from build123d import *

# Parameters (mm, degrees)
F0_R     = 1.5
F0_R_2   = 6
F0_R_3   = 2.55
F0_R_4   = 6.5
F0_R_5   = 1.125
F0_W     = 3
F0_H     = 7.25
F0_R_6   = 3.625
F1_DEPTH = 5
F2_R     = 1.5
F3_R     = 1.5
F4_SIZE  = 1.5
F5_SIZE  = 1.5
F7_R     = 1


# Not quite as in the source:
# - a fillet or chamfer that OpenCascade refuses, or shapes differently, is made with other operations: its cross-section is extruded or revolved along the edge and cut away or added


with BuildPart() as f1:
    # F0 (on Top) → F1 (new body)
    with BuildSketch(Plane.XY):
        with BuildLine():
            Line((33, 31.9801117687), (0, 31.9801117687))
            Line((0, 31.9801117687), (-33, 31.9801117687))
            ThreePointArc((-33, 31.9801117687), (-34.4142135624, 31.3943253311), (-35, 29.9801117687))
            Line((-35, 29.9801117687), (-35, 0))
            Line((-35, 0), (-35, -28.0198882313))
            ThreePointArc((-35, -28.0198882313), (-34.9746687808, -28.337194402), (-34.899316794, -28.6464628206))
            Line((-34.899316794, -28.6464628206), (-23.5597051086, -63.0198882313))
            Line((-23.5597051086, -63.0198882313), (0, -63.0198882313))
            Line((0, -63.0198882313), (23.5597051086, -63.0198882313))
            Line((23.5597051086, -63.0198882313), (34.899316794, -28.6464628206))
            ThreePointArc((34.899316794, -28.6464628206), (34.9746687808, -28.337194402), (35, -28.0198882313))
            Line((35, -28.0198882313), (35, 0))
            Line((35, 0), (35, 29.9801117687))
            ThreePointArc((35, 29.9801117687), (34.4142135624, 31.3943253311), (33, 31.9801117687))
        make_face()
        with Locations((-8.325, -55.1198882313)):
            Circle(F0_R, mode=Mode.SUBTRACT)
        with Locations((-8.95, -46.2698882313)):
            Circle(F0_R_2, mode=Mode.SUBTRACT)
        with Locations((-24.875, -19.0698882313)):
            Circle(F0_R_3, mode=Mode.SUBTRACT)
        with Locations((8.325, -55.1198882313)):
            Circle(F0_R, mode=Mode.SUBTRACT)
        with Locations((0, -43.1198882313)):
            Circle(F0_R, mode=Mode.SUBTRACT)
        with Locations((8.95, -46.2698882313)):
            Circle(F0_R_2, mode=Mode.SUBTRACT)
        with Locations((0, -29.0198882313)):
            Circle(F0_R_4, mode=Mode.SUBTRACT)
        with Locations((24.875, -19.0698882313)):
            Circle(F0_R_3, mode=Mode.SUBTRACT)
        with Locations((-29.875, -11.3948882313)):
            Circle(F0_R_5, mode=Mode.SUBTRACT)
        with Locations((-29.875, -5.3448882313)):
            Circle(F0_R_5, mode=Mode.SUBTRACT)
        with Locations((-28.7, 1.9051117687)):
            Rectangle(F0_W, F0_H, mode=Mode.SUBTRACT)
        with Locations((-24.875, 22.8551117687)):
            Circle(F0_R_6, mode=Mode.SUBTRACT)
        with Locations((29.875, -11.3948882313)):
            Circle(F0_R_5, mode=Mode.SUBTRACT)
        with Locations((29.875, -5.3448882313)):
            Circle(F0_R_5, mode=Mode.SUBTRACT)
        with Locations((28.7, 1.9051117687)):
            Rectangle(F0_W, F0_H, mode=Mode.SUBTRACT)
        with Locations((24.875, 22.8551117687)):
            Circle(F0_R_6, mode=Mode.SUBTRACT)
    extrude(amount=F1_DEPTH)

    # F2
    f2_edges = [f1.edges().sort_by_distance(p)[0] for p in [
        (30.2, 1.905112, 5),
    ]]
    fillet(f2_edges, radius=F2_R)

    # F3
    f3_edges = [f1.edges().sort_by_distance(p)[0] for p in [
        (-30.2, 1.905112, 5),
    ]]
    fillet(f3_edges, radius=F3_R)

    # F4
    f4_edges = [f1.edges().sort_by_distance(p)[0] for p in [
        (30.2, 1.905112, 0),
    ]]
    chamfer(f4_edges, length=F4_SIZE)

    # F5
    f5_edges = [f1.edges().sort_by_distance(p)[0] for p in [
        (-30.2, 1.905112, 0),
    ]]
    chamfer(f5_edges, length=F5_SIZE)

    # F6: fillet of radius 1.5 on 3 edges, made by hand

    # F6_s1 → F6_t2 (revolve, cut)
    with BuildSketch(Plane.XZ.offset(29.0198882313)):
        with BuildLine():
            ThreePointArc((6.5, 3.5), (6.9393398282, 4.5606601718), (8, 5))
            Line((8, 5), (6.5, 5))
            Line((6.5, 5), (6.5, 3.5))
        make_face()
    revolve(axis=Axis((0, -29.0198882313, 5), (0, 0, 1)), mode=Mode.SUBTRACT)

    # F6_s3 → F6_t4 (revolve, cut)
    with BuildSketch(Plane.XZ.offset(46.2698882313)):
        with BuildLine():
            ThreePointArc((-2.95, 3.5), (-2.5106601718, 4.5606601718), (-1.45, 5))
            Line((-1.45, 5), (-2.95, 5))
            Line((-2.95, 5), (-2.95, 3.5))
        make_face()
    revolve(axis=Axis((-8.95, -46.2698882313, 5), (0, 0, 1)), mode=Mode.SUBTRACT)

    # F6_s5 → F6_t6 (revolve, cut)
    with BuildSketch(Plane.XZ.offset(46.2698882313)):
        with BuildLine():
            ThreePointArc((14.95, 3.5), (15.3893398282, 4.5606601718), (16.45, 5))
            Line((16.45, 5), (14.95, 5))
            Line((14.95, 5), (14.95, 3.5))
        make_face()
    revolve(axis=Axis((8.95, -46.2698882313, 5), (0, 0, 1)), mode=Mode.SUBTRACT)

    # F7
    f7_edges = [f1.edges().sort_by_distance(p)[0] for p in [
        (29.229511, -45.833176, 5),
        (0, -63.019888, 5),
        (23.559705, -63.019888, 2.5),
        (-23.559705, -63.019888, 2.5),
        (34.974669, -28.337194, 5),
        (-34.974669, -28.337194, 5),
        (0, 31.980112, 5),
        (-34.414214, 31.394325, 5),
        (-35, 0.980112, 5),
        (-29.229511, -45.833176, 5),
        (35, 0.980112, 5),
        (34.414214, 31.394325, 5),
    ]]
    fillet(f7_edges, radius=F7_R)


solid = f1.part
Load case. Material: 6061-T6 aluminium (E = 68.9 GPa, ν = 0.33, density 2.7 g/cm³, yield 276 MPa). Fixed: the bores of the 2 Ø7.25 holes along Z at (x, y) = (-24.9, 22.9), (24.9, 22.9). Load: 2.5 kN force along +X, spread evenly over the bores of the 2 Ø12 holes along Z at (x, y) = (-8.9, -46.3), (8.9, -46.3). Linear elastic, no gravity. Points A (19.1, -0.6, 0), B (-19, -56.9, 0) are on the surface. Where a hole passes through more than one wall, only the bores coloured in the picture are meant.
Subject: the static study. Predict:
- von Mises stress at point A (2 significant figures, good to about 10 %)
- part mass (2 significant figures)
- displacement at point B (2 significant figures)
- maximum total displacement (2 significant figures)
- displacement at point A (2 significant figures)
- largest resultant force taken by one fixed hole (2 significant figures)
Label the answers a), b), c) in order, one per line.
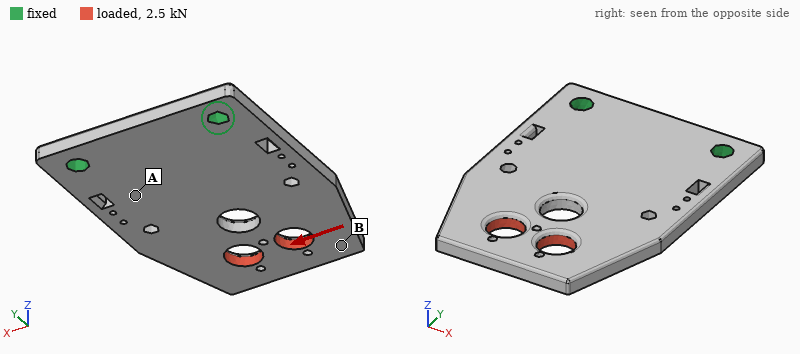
a) 24 MPa
b) 76 g
c) 84 µm
d) 93 µm
e) 15 µm
f) 3.5 kN
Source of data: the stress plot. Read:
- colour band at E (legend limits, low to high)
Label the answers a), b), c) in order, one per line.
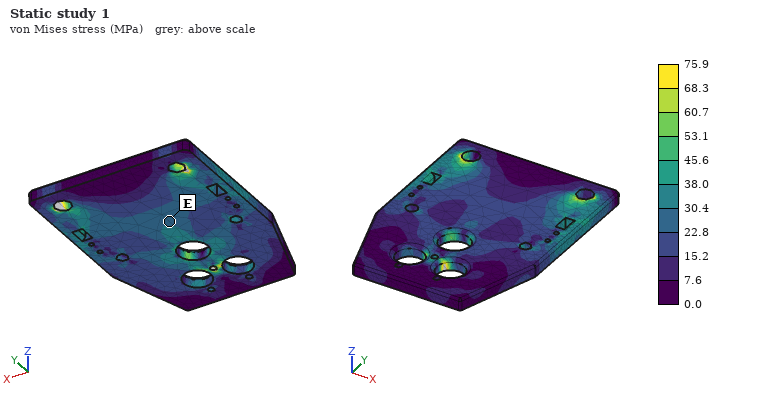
a) 22.8 to 30.4 MPa
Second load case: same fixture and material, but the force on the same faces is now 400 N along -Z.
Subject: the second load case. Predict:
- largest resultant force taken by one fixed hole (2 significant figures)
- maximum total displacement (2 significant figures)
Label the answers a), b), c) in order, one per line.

a) 200 N
b) 1.3 mm
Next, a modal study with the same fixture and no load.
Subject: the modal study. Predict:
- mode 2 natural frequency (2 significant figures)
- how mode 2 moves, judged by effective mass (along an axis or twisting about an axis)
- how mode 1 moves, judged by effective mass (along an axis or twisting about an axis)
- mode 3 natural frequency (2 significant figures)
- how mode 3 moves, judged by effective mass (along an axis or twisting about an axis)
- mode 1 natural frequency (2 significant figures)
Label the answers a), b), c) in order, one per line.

a) 1900 Hz
b) twisting about Y
c) along Z
d) 3300 Hz
e) along Z
f) 640 Hz
